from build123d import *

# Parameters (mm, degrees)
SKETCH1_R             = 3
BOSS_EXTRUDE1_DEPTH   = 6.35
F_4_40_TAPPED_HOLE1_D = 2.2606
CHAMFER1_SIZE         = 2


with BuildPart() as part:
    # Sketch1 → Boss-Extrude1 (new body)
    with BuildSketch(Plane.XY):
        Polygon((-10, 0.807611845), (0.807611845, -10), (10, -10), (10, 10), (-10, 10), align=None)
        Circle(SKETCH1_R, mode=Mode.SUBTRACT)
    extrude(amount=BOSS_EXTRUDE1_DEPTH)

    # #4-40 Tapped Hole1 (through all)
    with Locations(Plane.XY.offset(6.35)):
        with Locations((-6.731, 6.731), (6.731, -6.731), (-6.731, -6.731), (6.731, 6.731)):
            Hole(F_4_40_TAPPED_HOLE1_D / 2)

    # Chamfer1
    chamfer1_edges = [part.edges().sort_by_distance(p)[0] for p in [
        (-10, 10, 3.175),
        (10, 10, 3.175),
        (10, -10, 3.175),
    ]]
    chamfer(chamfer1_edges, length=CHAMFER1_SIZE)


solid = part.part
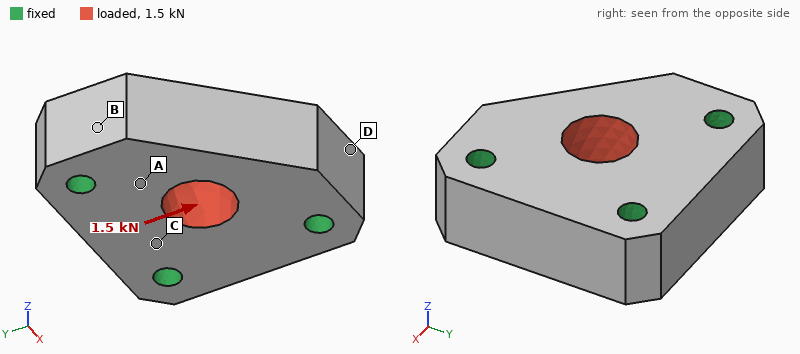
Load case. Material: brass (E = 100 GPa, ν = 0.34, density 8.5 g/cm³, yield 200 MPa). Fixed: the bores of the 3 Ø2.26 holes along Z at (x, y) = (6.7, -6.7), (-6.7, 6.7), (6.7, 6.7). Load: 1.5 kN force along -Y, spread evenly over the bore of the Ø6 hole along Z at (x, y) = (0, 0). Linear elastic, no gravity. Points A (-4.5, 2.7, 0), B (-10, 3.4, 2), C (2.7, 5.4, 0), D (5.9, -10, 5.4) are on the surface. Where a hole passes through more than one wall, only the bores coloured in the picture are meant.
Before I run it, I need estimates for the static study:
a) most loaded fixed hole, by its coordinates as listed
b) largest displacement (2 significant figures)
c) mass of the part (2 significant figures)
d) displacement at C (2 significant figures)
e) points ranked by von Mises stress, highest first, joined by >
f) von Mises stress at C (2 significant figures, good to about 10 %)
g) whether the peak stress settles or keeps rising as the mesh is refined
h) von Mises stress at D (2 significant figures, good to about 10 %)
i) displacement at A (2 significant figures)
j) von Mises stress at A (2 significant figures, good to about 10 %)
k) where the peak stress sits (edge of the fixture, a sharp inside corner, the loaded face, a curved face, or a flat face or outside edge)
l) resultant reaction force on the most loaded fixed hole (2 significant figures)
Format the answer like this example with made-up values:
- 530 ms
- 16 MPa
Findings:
- (-6.7, 6.7)
- 2.3 µm
- 16 g
- 0.83 µm
- A > C > D > B
- 14 MPa
- keeps rising
- 8.7 MPa
- 0.91 µm
- 17 MPa
- edge of the fixture
- 650 N
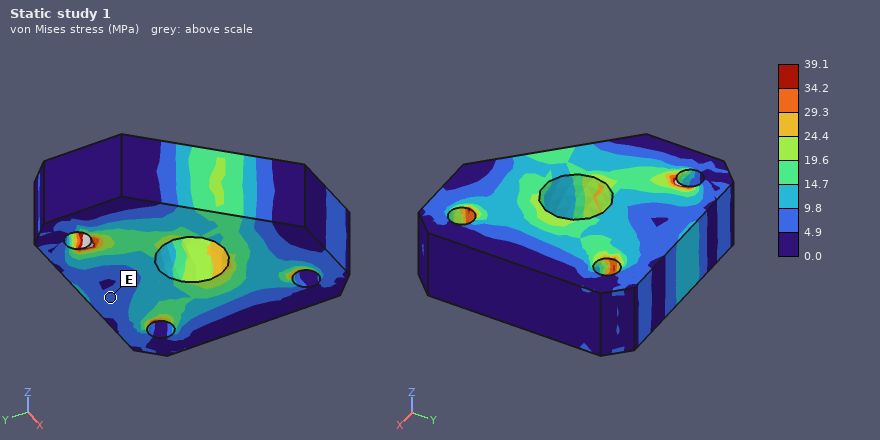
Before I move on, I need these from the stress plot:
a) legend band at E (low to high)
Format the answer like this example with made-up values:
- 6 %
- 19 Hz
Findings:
- 4.9 to 9.8 MPa
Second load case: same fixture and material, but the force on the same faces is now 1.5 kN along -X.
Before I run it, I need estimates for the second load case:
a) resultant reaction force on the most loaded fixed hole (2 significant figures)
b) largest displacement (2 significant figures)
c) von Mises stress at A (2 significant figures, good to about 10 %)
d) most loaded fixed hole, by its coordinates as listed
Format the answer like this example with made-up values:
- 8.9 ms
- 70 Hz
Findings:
- 650 N
- 2.3 µm
- 13 MPa
- (6.7, -6.7)
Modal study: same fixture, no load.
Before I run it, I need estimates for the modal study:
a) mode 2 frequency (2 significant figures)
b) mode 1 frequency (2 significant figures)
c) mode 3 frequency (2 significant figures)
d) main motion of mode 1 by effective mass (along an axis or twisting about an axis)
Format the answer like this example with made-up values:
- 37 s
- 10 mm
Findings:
- 56 kHz
- 35 kHz
- 59 kHz
- along Z
